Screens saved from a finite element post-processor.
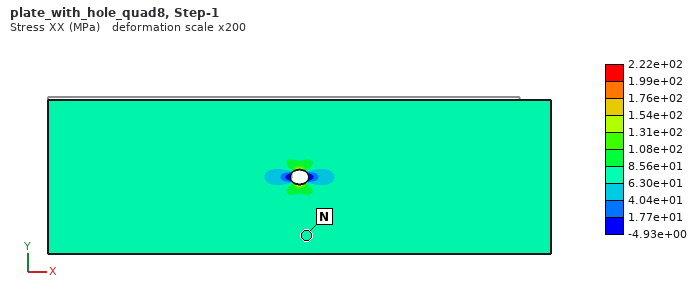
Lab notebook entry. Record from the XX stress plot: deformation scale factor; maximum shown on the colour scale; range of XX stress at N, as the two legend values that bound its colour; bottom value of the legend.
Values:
200
2.22e+02 MPa
6.30e+01 to 8.56e+01 MPa
-4.93e+00 MPa
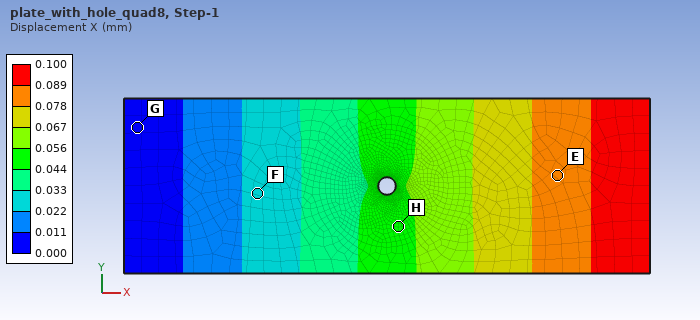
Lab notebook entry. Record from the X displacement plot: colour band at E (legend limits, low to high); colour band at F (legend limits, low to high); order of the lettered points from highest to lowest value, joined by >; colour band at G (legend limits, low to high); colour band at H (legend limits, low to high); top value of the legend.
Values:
0.078 to 0.089 mm
0.022 to 0.033 mm
E > H > F > G
0.000 to 0.011 mm
0.044 to 0.056 mm
0.100 mm
